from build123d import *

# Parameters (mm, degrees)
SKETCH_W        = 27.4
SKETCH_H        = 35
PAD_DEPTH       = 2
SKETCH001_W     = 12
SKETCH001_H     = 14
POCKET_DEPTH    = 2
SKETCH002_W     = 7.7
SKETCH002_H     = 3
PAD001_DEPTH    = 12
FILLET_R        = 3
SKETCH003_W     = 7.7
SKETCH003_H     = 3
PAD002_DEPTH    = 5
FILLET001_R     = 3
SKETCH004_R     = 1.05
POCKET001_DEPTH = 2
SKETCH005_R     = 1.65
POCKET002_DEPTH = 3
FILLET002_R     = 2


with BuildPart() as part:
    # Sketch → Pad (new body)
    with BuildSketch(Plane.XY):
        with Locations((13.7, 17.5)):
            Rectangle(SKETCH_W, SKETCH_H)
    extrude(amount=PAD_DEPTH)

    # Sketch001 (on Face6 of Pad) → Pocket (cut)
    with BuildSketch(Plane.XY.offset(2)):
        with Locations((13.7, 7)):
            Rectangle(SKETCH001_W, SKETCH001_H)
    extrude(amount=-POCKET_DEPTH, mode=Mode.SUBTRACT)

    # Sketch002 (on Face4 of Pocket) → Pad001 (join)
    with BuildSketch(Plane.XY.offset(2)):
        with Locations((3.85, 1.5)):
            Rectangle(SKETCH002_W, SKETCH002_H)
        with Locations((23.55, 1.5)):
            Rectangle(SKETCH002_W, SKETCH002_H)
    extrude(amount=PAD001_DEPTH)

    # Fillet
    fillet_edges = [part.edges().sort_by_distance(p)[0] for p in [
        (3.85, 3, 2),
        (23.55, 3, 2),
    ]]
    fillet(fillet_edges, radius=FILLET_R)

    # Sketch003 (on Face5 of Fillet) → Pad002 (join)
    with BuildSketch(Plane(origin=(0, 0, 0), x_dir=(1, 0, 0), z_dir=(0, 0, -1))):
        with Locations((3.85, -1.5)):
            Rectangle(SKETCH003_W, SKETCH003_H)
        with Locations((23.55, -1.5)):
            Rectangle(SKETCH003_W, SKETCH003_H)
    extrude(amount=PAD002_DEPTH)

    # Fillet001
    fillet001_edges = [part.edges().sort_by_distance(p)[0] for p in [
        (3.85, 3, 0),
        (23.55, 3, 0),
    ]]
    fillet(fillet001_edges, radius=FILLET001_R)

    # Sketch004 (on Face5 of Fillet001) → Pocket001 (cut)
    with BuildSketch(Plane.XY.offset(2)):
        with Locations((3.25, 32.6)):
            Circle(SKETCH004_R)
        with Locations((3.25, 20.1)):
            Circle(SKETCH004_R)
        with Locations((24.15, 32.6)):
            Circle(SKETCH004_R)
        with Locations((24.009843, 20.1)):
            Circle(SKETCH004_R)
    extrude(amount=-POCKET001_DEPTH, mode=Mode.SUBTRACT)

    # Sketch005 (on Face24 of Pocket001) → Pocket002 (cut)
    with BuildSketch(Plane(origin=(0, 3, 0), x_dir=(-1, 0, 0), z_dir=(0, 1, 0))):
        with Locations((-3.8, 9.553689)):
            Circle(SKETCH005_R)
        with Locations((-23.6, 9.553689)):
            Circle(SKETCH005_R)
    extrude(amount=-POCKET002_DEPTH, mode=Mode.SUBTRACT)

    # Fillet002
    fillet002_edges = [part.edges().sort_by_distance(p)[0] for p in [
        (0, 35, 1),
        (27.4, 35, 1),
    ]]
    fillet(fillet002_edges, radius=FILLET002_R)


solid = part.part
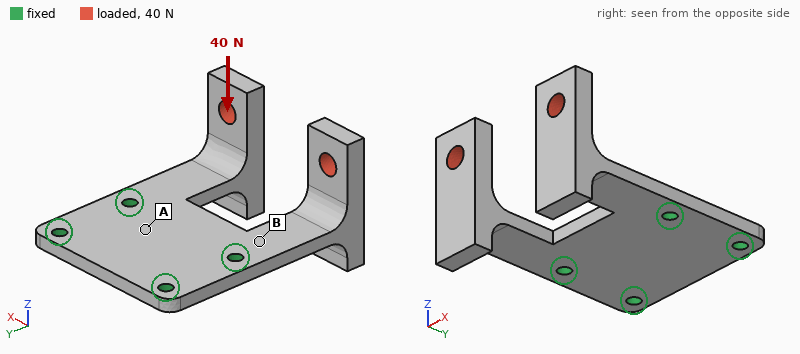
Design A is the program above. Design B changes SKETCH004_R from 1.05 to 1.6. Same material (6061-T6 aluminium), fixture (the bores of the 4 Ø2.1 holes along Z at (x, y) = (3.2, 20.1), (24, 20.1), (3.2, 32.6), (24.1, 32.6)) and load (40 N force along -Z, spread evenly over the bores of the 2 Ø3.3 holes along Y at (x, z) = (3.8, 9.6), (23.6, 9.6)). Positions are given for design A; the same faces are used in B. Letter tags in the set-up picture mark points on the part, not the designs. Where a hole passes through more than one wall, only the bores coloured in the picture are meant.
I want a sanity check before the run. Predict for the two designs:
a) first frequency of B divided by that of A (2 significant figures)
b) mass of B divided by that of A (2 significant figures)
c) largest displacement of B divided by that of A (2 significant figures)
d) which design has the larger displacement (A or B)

1.0
0.98
0.92
A
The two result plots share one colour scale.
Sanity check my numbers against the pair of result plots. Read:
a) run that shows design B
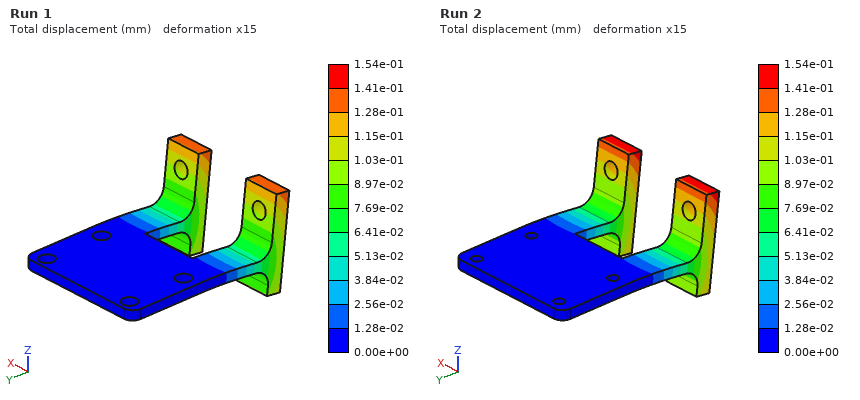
Run 1
